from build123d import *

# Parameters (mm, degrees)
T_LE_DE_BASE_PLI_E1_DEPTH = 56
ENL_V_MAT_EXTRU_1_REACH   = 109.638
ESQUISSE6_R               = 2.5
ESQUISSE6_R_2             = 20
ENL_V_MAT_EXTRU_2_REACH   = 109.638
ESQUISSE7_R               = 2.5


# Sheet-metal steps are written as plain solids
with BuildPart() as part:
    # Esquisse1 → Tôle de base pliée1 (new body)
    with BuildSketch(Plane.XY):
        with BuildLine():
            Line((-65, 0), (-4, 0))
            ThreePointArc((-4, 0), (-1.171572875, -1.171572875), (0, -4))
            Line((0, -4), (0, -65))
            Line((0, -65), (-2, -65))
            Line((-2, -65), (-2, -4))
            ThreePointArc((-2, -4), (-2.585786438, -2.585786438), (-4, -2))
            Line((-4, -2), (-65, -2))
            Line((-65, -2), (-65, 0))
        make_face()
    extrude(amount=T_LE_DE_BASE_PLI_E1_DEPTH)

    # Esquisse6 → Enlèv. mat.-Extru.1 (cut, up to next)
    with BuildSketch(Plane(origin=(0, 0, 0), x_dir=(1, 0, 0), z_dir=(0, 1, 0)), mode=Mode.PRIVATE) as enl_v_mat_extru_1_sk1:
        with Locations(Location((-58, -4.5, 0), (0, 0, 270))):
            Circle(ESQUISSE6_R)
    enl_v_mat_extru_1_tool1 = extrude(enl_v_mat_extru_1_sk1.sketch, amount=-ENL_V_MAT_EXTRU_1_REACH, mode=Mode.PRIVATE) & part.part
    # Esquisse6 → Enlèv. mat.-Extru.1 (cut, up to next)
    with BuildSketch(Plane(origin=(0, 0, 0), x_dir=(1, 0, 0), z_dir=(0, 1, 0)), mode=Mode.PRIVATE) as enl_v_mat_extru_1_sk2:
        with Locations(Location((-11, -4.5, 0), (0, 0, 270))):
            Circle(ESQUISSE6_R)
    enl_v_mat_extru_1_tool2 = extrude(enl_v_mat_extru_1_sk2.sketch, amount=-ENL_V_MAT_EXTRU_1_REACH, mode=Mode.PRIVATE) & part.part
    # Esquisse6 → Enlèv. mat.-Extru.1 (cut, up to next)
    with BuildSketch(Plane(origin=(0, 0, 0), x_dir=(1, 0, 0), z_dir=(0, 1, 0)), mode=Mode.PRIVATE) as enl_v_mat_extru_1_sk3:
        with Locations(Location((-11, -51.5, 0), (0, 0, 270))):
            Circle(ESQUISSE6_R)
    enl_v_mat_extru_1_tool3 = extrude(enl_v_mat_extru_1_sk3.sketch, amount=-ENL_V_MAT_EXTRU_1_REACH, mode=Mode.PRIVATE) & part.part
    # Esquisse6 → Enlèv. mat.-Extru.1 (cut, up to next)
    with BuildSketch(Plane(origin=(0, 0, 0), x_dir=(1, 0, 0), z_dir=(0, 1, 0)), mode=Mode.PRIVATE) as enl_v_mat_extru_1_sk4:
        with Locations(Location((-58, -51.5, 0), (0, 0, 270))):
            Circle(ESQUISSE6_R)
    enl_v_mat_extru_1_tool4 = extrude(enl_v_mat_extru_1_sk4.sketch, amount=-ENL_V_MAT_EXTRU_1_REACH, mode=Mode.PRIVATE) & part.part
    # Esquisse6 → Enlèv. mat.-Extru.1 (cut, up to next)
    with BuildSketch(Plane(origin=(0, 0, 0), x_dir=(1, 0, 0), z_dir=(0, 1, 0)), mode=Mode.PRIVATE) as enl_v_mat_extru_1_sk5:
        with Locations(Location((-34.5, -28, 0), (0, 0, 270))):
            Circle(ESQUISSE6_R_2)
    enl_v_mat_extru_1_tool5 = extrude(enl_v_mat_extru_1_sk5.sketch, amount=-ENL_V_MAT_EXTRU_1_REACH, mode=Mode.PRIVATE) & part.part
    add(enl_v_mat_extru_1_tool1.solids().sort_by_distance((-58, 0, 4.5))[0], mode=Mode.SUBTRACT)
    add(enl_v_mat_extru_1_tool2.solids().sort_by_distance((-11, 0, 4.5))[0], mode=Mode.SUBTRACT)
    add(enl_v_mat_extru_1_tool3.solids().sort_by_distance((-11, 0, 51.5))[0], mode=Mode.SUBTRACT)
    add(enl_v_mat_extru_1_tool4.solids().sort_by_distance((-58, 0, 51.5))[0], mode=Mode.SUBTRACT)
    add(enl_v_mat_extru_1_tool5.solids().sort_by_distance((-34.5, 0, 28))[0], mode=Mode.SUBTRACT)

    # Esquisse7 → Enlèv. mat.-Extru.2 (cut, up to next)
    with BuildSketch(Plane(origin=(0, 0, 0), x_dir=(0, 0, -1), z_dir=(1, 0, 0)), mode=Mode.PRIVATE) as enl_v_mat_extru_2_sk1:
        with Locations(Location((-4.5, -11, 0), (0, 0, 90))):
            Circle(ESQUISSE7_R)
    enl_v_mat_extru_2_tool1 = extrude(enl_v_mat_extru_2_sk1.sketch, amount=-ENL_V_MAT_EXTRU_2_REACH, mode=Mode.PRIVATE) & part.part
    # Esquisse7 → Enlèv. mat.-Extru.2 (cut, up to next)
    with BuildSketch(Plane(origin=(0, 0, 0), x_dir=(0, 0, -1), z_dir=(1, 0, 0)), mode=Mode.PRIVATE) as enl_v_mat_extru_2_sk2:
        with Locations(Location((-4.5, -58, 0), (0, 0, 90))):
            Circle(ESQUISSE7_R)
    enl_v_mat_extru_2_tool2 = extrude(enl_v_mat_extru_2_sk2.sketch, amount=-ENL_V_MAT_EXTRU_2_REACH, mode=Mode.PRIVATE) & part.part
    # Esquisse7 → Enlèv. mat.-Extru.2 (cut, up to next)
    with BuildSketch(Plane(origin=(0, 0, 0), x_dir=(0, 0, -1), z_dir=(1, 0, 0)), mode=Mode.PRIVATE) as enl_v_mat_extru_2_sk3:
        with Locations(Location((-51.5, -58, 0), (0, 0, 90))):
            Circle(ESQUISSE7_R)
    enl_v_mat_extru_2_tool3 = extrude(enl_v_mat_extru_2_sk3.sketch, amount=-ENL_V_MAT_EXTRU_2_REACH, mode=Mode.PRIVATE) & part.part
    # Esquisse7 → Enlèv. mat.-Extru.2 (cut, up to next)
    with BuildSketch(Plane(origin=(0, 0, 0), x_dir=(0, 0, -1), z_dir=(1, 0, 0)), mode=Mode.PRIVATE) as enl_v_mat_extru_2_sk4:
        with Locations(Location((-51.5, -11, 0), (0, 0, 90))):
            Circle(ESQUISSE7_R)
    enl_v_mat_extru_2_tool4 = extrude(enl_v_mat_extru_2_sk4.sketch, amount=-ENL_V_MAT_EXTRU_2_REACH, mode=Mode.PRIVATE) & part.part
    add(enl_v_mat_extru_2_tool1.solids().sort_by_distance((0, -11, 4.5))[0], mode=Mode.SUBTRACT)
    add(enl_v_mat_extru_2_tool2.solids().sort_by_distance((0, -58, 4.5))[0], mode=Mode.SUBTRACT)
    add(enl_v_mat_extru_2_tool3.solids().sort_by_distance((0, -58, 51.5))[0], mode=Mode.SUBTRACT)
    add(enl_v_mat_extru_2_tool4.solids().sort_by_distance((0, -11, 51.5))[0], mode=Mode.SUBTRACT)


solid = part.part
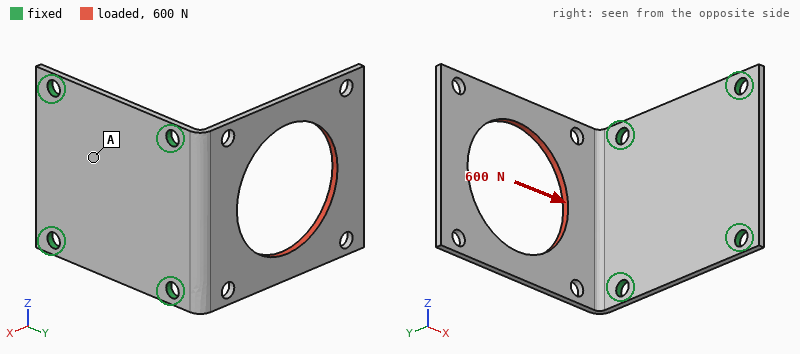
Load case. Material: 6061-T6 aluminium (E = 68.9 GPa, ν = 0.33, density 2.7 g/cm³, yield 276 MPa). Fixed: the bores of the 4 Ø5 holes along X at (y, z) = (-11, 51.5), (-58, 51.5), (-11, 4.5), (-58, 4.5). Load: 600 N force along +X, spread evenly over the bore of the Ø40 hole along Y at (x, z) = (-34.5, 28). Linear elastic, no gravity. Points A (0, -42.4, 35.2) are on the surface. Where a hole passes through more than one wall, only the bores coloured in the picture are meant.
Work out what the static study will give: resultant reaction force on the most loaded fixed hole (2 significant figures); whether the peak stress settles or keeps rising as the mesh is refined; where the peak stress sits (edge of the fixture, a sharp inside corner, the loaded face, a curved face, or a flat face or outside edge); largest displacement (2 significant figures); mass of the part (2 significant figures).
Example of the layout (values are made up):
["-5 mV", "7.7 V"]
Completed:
["310 N", "keeps rising", "edge of the fixture", "0.71 mm", "31 g"]
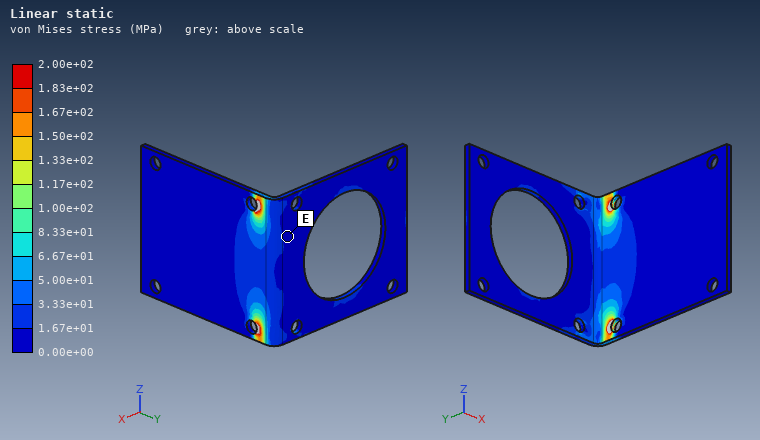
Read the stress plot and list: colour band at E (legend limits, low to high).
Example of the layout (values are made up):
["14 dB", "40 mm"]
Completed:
["0.00e+00 to 1.67e+01 MPa"]
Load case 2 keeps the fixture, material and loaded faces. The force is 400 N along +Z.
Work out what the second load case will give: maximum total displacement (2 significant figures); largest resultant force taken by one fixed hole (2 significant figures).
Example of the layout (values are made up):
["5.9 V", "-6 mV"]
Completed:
["0.33 mm", "360 N"]
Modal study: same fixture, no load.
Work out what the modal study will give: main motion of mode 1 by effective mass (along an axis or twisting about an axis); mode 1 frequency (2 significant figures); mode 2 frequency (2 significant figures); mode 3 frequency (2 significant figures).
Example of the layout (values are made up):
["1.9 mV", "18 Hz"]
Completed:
["along Y", "310 Hz", "820 Hz", "1900 Hz"]
